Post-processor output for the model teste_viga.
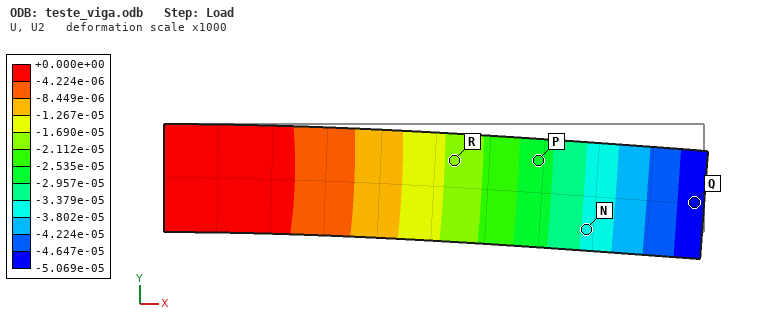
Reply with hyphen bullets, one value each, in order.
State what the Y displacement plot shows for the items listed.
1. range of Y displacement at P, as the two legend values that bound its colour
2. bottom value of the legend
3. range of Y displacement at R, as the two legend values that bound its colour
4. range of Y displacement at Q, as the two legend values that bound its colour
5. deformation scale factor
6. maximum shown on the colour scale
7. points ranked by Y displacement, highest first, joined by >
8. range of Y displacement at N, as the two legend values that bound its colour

- -2.957e-05 to -2.535e-05
- -5.069e-05
- -2.112e-05 to -1.690e-05
- -5.069e-05 to -4.647e-05
- 1000
- +0.000e+00
- R > P > N > Q
- -3.802e-05 to -3.379e-05
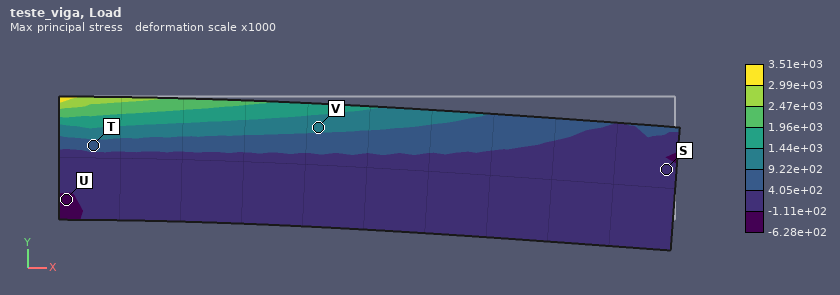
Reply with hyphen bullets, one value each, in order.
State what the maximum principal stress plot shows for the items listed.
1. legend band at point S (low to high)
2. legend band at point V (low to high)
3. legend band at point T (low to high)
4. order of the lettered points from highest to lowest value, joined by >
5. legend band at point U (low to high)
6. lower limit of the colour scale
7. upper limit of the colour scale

- -1.11e+02 to 4.05e+02
- 9.22e+02 to 1.44e+03
- 4.05e+02 to 9.22e+02
- V > T > S > U
- -6.28e+02 to -1.11e+02
- -6.28e+02
- 3.51e+03
